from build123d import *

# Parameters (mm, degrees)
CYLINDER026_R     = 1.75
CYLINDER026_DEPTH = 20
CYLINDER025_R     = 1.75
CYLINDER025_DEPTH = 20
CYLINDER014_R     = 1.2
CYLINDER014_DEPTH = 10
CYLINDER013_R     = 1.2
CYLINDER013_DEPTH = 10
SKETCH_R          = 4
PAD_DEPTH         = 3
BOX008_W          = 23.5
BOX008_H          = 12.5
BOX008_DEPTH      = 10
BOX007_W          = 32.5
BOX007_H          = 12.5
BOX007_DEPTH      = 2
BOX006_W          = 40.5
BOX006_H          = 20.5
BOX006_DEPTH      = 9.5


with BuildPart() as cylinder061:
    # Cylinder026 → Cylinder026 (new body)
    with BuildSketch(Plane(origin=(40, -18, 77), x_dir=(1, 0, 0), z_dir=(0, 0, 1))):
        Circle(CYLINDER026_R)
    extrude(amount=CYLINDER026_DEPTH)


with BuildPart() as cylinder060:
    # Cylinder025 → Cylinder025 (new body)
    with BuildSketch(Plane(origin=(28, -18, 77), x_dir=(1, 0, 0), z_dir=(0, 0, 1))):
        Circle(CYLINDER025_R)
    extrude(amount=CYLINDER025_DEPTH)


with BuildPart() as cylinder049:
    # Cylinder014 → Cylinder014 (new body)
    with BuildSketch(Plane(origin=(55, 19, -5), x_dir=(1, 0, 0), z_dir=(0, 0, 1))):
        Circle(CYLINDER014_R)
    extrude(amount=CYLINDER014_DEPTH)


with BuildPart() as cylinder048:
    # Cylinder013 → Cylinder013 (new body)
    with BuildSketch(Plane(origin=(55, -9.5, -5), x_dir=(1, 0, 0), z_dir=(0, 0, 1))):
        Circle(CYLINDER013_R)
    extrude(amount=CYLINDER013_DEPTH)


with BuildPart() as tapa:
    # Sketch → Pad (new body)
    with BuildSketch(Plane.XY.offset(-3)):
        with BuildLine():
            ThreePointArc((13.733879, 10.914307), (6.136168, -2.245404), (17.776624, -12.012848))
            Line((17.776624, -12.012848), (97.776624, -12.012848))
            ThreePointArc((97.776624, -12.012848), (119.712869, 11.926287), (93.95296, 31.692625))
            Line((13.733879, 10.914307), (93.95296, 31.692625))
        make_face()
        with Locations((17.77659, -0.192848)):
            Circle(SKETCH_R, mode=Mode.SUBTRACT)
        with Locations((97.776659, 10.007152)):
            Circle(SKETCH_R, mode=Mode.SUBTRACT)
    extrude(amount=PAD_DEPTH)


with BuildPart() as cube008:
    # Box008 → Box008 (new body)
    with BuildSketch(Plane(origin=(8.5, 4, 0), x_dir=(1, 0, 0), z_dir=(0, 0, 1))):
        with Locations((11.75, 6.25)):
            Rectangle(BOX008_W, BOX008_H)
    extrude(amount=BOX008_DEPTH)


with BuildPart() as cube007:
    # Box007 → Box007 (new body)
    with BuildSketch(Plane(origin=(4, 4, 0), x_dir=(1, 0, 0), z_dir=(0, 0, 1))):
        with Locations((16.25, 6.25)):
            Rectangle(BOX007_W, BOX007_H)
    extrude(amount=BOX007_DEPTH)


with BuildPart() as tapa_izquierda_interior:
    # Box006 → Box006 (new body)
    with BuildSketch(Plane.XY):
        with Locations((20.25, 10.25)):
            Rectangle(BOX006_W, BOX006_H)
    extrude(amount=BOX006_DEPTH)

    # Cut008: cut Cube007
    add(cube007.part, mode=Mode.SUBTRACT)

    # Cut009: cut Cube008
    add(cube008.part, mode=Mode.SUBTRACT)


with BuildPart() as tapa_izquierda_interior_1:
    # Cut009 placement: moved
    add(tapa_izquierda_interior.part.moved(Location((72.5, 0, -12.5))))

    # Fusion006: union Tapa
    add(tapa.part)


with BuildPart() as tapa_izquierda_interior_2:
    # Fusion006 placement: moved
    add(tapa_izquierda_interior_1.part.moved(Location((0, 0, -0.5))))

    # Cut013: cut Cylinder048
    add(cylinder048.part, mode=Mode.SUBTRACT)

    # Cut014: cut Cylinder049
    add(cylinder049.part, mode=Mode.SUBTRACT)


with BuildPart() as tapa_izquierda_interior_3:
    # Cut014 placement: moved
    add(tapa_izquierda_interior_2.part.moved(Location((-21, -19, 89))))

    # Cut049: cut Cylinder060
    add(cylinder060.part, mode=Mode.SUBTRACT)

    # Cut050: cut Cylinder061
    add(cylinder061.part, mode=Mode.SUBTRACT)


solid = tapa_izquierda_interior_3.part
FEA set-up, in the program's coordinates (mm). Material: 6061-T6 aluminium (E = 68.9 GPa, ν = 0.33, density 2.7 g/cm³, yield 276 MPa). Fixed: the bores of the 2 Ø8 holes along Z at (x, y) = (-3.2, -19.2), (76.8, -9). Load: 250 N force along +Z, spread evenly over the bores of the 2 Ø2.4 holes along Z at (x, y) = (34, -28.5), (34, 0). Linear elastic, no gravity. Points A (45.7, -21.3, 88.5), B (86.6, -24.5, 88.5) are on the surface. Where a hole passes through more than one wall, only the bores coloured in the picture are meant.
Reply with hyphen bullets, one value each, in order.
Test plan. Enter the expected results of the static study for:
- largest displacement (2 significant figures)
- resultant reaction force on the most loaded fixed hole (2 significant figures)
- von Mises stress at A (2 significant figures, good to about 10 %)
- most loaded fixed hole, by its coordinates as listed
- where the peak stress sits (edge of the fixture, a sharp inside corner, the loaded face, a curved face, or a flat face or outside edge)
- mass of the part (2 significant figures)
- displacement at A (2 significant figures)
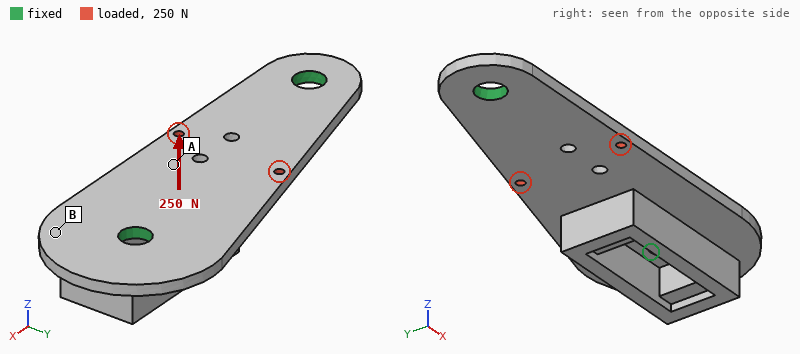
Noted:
- 95 µm
- 170 N
- 11 MPa
- (76.8, -9)
- the loaded face
- 42 g
- 53 µm
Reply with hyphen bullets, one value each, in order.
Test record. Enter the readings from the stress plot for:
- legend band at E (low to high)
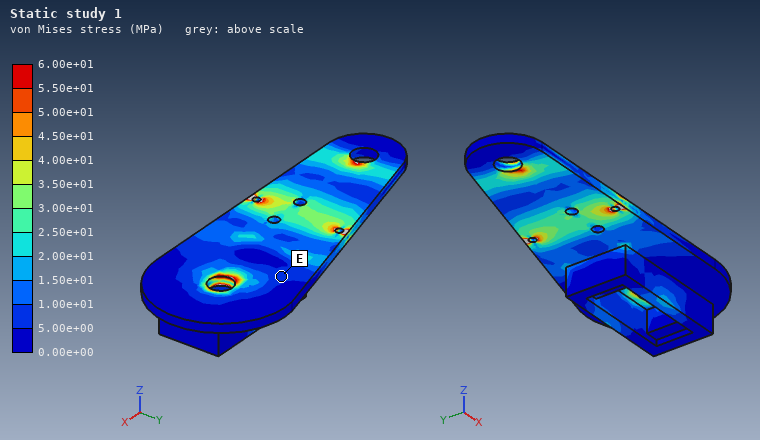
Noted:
- 5.00e+00 to 1.00e+01 MPa
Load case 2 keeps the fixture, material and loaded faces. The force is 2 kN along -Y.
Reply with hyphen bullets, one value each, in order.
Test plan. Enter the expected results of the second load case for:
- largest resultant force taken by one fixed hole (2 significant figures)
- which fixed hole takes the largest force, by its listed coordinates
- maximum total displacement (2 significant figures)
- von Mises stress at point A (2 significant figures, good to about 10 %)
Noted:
- 1.1 kN
- (-3.2, -19.2)
- 40 µm
- 28 MPa
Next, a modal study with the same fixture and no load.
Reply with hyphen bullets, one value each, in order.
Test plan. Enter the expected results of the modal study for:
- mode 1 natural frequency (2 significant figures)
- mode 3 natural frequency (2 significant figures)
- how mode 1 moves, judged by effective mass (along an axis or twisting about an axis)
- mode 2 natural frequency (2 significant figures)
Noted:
- 3100 Hz
- 6500 Hz
- along Z
- 4800 Hz
